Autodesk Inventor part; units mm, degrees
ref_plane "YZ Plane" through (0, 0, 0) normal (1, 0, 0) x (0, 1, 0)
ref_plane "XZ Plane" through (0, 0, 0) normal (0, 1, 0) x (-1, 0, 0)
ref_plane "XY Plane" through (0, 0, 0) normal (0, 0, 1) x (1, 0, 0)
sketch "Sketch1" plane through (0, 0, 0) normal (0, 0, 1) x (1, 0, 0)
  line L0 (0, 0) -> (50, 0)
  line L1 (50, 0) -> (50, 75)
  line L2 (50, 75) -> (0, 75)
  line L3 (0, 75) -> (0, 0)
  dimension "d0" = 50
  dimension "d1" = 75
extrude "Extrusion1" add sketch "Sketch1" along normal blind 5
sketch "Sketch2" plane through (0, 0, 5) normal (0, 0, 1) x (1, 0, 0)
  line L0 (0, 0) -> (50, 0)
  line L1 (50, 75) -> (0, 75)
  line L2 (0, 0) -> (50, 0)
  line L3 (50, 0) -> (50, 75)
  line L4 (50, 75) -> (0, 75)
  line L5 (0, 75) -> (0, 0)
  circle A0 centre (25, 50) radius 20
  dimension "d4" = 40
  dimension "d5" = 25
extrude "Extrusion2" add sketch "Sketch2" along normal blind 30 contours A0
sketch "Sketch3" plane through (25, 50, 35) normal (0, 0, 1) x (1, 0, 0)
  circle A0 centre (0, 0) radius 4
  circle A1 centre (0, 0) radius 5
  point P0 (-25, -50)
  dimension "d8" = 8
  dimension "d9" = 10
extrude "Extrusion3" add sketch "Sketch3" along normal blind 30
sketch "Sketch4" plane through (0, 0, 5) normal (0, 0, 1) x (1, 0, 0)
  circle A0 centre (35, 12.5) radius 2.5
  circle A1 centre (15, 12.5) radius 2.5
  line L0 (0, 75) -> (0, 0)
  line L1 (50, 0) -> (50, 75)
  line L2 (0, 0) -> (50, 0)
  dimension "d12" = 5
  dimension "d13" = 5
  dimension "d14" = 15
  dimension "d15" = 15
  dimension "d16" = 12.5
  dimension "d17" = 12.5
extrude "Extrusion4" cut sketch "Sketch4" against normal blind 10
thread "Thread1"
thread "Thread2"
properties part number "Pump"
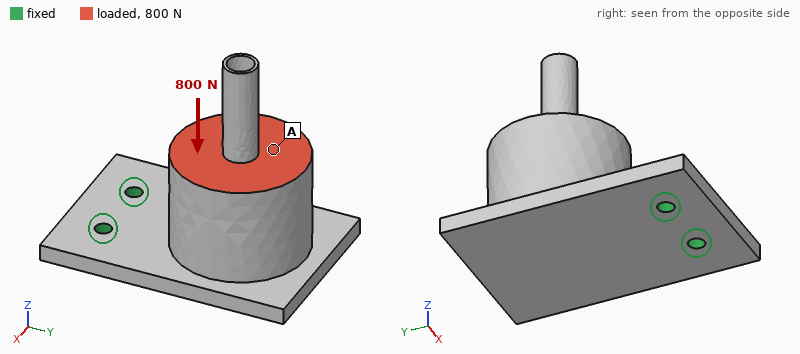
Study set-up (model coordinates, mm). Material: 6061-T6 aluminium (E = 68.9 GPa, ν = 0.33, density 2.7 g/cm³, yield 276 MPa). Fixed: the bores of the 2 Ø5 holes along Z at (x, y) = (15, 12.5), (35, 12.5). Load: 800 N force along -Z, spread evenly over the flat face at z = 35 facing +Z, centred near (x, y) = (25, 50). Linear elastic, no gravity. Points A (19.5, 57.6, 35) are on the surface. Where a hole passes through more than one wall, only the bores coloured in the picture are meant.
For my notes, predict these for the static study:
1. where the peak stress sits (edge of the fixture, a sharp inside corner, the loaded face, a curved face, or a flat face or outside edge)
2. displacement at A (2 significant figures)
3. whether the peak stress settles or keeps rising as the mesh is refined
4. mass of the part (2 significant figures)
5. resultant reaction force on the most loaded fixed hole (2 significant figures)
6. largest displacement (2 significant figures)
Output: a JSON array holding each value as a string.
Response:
["edge of the fixture", "0.61 mm", "keeps rising", "150 g", "400 N", "0.89 mm"]
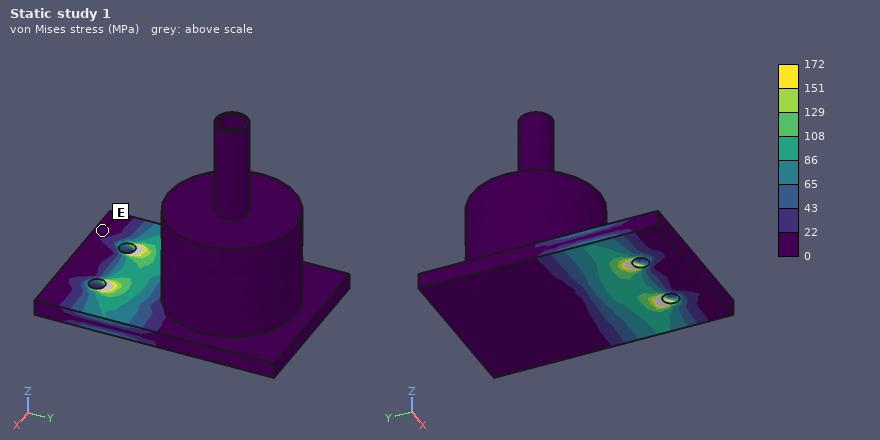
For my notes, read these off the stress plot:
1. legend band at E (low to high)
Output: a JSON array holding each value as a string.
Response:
["0 to 22 MPa"]
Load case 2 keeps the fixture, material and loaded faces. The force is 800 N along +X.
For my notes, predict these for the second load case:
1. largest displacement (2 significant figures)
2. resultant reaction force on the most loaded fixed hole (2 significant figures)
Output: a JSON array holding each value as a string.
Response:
["0.32 mm", "1.6 kN"]
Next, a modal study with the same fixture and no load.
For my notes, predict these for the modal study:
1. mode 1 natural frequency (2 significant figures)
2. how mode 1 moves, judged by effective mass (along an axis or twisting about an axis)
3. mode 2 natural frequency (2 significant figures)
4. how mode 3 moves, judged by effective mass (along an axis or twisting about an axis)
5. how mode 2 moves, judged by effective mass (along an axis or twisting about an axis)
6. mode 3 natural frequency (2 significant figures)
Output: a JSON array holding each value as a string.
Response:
["510 Hz", "along Z", "1400 Hz", "along X", "along X", "3800 Hz"]
